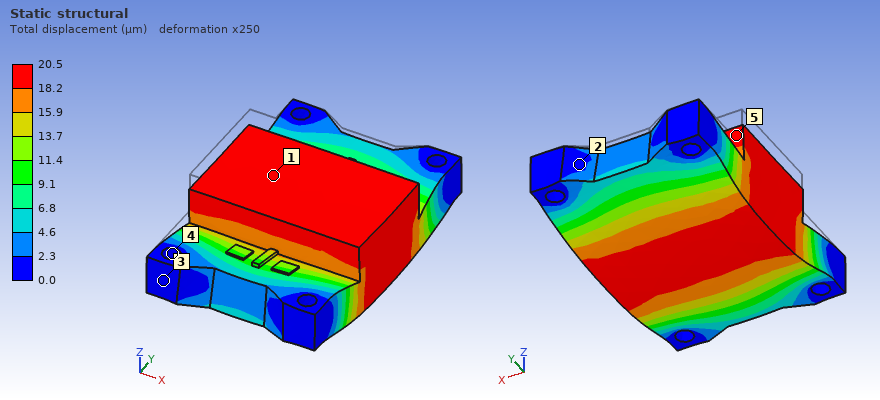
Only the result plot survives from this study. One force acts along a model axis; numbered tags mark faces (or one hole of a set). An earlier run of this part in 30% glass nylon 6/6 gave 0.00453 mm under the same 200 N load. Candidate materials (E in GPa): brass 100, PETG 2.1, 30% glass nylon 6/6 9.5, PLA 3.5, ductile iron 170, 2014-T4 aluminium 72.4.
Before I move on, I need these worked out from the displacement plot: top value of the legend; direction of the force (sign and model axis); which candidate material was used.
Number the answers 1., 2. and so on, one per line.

1. 20.5 µm
2. -Z
3. PETG
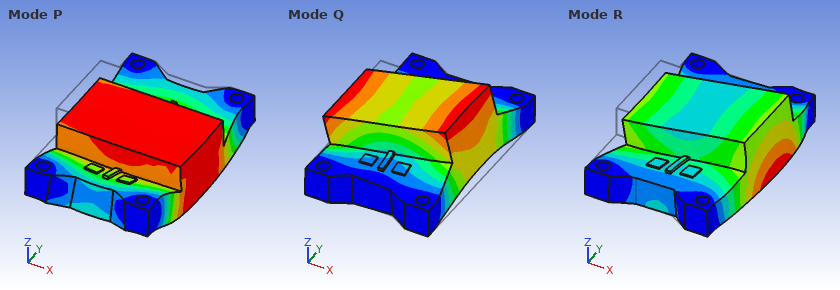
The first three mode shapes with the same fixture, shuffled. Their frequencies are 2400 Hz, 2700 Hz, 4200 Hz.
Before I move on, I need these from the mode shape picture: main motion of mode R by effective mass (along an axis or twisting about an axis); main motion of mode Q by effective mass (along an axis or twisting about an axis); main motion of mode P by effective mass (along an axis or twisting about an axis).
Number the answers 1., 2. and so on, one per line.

1. along X
2. along X
3. along Z
